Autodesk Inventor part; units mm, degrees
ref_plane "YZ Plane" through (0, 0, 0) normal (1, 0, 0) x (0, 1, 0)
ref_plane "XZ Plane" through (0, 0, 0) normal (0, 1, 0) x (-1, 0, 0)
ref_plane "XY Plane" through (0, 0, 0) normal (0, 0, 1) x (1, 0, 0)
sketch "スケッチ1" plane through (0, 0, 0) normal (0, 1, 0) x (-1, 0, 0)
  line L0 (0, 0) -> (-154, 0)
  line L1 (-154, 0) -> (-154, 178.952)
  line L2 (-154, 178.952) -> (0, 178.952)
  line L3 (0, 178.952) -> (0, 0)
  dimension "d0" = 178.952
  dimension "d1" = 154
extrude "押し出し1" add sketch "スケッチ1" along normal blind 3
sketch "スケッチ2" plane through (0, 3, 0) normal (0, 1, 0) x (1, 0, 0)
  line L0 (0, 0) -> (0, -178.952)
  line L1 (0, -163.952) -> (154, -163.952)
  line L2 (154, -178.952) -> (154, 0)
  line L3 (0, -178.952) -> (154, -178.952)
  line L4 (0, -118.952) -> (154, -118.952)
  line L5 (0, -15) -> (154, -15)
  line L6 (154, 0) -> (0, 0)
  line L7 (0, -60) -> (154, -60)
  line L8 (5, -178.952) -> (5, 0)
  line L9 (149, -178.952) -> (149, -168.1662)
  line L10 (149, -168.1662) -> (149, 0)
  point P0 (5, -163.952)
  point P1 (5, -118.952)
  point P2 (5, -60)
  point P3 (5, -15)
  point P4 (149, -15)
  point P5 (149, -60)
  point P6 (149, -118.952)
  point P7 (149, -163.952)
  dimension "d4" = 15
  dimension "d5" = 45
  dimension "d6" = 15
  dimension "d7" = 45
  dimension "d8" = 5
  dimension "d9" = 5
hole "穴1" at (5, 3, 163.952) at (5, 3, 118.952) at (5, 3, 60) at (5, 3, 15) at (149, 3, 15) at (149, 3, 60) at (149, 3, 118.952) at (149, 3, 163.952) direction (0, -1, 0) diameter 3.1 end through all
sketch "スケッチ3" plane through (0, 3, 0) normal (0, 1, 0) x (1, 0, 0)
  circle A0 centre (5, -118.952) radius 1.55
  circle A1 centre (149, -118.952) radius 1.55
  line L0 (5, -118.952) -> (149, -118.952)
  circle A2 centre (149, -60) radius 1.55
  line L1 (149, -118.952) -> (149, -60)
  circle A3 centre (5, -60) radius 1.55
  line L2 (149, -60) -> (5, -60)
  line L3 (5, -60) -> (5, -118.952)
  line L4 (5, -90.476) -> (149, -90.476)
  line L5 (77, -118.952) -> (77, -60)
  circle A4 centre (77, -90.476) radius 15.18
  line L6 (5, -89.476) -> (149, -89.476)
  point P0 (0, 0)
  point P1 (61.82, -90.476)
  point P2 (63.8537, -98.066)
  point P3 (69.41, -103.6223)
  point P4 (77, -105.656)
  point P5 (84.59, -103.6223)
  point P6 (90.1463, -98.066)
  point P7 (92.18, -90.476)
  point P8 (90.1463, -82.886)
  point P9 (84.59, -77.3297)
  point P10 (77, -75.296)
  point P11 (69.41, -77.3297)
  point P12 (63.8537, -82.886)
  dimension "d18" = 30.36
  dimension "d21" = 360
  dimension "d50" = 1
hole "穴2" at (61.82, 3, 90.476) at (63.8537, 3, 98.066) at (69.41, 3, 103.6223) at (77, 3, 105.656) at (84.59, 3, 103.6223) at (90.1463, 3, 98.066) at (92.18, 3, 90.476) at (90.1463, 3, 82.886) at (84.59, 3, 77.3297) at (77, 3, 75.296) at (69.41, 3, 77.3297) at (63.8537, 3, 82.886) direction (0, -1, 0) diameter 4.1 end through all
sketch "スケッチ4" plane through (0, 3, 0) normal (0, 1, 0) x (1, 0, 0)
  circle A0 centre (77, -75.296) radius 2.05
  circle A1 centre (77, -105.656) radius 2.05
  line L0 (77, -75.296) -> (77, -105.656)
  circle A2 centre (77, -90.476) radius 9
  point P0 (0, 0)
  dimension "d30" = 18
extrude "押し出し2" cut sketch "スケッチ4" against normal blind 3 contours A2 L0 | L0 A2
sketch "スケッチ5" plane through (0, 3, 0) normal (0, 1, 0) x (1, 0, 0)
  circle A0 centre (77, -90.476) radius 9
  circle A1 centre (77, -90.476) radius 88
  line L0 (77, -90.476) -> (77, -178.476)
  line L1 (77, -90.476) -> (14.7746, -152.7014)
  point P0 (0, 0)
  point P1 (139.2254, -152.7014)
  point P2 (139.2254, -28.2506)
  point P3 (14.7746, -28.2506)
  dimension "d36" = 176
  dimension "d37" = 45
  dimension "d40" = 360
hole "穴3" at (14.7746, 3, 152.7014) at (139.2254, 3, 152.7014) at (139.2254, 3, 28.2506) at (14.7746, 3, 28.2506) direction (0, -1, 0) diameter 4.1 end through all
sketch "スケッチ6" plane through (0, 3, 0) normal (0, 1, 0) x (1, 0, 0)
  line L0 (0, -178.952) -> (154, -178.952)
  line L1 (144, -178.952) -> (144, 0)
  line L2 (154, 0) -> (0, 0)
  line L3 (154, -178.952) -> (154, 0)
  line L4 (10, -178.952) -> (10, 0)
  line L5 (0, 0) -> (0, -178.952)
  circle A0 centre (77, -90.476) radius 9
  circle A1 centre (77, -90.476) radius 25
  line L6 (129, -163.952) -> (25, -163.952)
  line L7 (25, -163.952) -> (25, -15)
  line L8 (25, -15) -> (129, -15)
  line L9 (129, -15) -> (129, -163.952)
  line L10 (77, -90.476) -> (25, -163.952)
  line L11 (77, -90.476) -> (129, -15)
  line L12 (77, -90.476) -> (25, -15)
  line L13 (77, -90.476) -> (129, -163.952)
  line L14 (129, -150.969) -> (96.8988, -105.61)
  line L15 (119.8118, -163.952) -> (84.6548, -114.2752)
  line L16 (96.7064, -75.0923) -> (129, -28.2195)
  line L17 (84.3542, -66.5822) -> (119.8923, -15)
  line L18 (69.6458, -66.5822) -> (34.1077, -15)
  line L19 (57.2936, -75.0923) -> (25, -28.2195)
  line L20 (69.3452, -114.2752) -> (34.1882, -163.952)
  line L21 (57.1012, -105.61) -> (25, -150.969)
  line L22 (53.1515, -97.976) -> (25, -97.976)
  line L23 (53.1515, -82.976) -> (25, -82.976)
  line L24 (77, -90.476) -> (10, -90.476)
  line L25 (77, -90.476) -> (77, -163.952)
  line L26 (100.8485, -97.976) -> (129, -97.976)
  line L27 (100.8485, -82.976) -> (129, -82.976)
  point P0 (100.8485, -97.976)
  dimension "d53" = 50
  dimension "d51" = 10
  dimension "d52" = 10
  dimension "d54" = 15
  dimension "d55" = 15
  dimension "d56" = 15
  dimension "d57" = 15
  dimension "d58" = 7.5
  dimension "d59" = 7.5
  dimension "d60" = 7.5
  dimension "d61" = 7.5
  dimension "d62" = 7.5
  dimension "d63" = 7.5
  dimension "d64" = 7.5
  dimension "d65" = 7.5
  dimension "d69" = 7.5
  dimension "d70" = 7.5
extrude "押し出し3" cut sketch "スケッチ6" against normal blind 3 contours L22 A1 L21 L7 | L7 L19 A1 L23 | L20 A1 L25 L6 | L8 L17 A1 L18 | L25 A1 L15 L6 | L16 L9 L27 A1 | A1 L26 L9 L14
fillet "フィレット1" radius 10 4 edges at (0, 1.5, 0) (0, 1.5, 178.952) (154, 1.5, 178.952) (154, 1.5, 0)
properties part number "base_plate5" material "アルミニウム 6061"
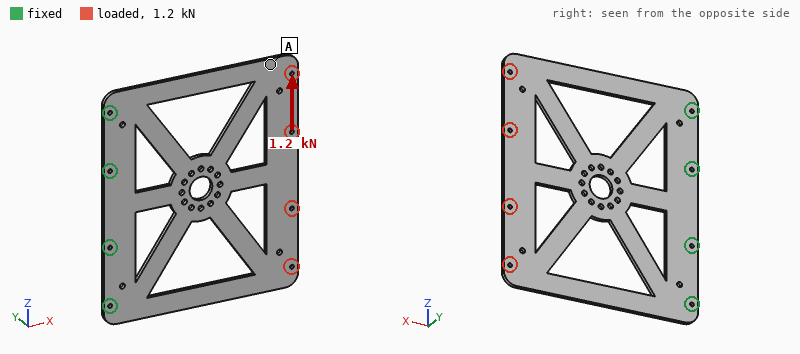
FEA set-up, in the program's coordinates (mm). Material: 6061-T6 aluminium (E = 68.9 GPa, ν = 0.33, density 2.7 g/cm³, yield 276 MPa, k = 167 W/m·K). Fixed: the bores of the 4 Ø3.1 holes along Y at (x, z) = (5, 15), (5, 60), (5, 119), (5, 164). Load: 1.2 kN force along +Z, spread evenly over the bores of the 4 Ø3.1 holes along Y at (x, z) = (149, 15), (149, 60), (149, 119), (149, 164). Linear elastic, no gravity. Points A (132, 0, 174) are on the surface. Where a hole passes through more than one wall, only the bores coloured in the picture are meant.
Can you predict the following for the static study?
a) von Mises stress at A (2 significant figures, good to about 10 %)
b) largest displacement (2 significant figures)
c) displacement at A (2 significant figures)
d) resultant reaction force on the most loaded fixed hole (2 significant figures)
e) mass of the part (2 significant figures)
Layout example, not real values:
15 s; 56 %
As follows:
6.2 MPa; 0.11 mm; 0.095 mm; 1.2 kN; 150 g
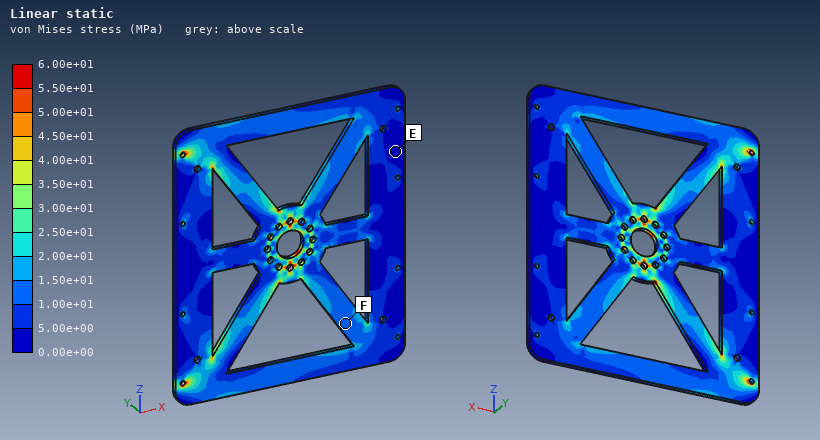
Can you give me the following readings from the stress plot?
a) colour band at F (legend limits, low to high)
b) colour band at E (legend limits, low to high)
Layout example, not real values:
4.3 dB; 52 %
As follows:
1.00e+01 to 1.50e+01 MPa; 0.00e+00 to 5.00e+00 MPa
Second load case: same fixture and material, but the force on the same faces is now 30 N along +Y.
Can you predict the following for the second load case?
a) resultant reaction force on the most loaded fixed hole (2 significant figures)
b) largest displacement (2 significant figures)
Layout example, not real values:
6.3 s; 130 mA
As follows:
8.0 N; 2.8 mm
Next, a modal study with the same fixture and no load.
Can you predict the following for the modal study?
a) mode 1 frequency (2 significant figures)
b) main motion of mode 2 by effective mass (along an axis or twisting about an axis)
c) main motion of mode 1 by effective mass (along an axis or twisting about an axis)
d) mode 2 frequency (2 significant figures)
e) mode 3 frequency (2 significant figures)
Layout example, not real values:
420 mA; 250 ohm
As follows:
82 Hz; twisting about X; along Y; 190 Hz; 510 Hz
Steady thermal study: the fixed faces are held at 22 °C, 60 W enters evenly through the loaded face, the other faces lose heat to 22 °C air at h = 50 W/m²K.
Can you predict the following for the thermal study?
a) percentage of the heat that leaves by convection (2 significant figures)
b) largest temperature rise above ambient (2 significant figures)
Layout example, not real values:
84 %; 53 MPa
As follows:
89 %; 77 K
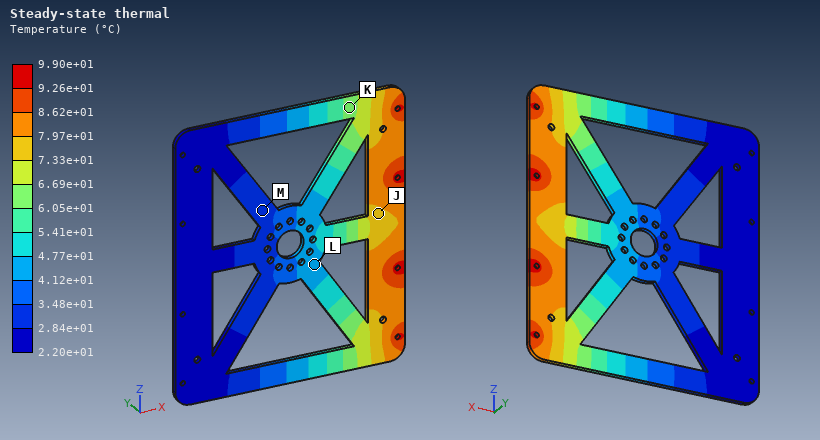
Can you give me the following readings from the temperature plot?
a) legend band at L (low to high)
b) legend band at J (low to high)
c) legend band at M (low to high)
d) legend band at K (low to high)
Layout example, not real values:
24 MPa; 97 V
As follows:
4.12e+01 to 4.77e+01 °C; 7.33e+01 to 7.97e+01 °C; 2.84e+01 to 3.48e+01 °C; 6.05e+01 to 6.69e+01 °C
